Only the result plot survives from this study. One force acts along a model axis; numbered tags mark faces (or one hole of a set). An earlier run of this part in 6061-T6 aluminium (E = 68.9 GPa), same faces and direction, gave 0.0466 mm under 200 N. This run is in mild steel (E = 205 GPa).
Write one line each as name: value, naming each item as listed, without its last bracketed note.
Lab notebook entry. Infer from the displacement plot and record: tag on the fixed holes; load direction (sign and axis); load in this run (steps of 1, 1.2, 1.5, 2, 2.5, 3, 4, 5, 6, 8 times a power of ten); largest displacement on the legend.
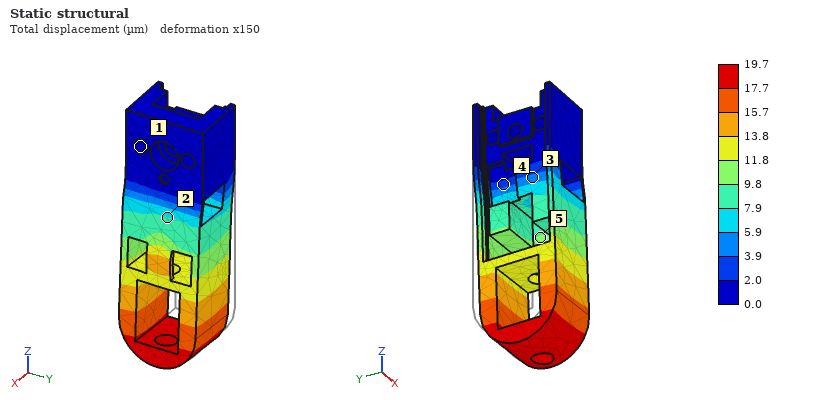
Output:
tag on the fixed holes: 1
load direction: +X
load in this run: 250 N
largest displacement on the legend: 19.7 µm
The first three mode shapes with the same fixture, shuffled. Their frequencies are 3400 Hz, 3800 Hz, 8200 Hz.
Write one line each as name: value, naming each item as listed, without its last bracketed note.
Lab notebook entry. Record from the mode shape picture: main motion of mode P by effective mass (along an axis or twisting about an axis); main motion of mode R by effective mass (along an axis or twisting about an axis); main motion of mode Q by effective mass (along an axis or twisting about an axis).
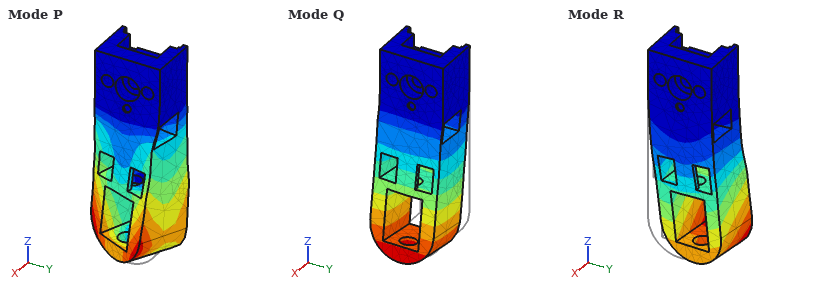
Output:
main motion of mode P by effective mass: twisting about Z
main motion of mode R by effective mass: along Y
main motion of mode Q by effective mass: along X
